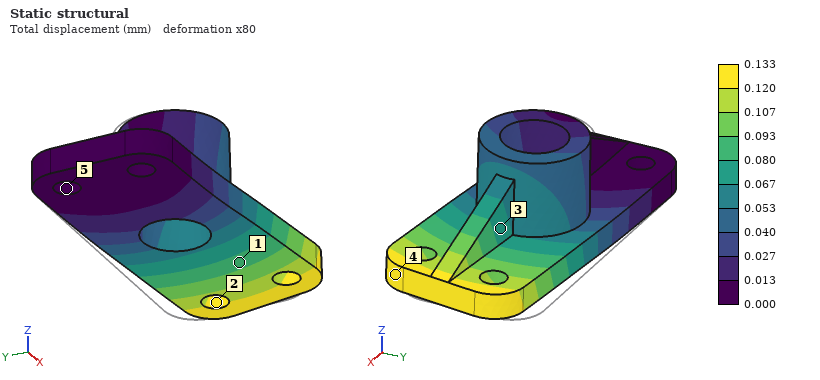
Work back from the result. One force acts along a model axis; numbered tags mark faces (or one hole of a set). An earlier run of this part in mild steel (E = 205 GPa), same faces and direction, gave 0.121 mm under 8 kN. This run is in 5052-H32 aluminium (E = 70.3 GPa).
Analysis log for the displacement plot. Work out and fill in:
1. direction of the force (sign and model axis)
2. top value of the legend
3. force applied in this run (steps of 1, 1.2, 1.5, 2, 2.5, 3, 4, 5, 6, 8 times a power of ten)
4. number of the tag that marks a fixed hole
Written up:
-Y
0.133 mm
3 kN
5
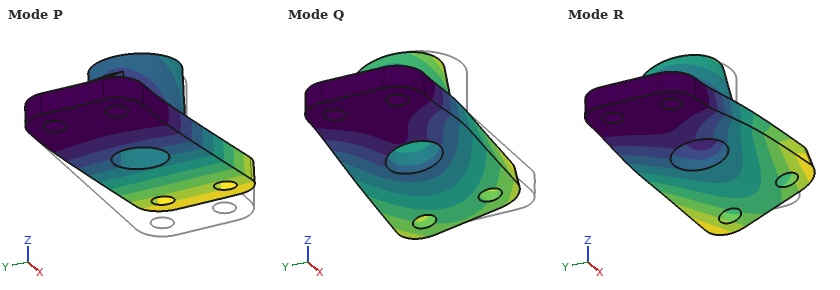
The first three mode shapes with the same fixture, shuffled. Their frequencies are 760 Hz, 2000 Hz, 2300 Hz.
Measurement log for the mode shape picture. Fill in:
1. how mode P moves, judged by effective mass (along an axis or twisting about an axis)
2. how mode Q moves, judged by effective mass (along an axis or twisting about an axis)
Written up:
along Z
along Y
